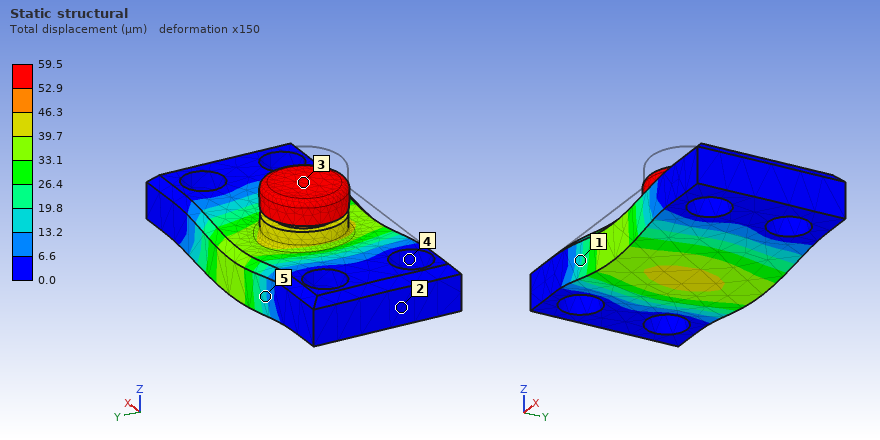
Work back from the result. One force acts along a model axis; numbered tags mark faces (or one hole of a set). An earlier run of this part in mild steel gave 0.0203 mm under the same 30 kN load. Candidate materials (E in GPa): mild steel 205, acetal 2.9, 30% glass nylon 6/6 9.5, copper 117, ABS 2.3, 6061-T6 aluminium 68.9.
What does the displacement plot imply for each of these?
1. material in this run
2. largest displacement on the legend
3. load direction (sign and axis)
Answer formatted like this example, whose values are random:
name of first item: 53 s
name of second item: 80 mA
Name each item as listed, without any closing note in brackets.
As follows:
material in this run: 6061-T6 aluminium
largest displacement on the legend: 59.5 µm
load direction: -Z
